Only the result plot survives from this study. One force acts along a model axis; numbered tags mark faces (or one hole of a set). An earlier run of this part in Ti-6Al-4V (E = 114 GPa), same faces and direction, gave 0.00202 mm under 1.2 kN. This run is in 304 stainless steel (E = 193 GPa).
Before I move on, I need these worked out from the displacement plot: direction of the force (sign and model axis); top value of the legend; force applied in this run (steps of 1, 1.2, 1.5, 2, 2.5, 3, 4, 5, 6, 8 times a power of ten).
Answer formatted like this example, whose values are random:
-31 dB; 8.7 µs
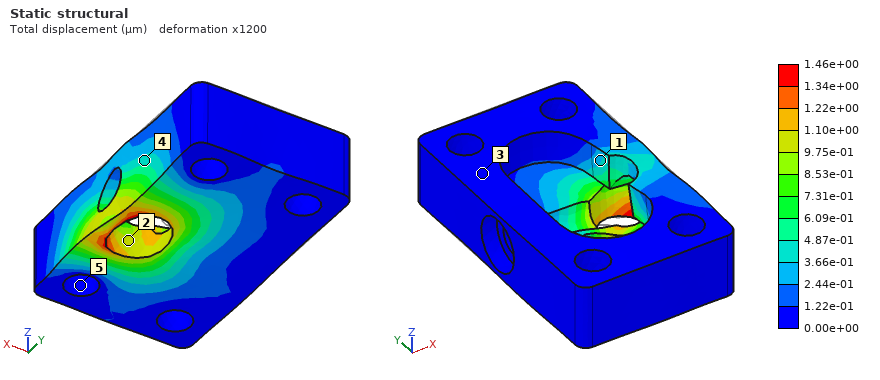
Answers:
-Y; 1.46e+00 µm; 1.5 kN
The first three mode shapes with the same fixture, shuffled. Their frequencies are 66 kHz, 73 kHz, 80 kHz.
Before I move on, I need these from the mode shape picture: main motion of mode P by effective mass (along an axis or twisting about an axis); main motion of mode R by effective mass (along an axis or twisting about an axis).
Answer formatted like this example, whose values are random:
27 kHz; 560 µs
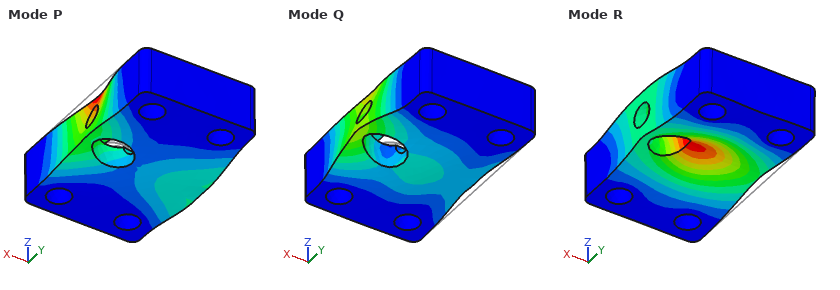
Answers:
along X; along Z
